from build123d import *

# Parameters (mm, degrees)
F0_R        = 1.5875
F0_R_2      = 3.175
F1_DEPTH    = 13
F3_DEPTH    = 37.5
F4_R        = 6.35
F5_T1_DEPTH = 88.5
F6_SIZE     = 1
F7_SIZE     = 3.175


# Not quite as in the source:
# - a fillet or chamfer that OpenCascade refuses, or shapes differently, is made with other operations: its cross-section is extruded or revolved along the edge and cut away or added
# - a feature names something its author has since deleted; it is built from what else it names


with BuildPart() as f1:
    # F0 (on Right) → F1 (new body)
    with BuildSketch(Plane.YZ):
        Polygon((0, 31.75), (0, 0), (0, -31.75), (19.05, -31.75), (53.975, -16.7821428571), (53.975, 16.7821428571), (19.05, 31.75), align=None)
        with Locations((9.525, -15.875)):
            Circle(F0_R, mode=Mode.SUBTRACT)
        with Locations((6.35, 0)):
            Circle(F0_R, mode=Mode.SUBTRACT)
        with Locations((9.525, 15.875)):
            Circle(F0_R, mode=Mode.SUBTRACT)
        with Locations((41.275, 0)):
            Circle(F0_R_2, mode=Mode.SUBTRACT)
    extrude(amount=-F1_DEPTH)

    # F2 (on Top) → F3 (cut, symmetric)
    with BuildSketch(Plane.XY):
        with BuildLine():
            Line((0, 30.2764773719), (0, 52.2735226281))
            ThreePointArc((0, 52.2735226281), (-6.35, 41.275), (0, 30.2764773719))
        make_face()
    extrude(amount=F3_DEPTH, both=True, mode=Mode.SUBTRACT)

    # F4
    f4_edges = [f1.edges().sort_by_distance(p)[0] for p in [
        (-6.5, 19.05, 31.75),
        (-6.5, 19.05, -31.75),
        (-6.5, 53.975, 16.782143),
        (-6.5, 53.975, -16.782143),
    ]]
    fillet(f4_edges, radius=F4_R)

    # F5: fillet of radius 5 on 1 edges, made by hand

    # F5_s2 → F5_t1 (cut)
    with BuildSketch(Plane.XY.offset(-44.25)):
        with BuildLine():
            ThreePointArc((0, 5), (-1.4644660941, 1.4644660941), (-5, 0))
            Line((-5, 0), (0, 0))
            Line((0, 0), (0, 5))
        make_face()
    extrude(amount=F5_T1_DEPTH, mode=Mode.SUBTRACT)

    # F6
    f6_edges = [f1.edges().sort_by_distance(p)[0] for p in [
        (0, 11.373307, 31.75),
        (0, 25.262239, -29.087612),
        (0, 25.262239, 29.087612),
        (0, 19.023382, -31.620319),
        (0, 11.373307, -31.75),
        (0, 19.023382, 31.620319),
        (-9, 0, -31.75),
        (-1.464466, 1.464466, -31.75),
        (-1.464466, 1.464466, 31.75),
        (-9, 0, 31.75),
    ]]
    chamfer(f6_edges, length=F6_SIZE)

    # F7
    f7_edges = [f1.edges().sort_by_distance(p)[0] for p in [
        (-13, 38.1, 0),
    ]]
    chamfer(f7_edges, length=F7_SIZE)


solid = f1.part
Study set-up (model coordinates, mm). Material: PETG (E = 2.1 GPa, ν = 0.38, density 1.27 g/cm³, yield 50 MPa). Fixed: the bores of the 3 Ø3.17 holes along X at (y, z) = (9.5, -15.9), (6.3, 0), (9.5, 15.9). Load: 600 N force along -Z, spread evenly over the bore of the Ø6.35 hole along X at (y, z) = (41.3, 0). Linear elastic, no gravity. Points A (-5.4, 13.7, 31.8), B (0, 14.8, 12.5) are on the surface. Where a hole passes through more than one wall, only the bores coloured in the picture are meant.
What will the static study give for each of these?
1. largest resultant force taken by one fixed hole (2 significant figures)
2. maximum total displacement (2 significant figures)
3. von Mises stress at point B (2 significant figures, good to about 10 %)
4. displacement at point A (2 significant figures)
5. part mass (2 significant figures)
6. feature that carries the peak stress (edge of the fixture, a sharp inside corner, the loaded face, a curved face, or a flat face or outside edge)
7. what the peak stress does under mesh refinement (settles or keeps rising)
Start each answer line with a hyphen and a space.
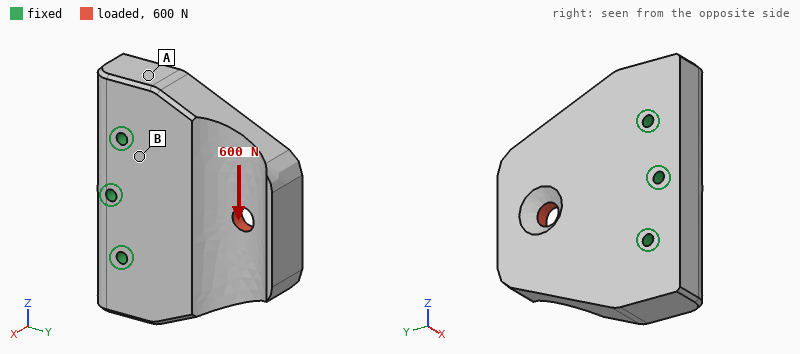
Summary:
- 630 N
- 0.13 mm
- 3.3 MPa
- 0.048 mm
- 41 g
- edge of the fixture
- keeps rising
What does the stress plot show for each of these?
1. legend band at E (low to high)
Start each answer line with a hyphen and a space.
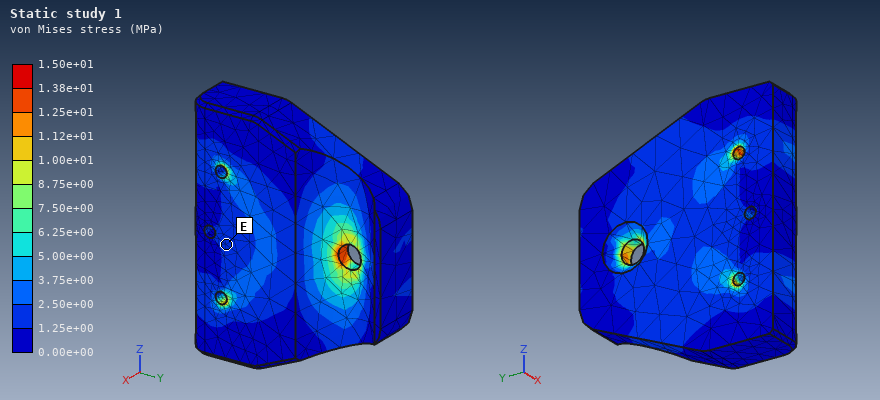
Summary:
- 1.25e+00 to 2.50e+00 MPa
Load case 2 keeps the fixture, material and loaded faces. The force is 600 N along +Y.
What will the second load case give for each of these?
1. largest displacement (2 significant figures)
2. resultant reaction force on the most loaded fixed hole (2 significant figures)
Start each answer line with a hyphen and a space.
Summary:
- 60 µm
- 220 N
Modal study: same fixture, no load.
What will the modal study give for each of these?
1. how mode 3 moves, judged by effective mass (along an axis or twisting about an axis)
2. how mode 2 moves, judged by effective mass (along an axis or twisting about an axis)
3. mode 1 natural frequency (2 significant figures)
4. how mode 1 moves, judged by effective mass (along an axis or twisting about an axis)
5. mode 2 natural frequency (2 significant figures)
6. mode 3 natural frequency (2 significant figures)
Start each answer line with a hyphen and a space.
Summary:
- along Z
- twisting about Y
- 1400 Hz
- along X
- 2800 Hz
- 3200 Hz
